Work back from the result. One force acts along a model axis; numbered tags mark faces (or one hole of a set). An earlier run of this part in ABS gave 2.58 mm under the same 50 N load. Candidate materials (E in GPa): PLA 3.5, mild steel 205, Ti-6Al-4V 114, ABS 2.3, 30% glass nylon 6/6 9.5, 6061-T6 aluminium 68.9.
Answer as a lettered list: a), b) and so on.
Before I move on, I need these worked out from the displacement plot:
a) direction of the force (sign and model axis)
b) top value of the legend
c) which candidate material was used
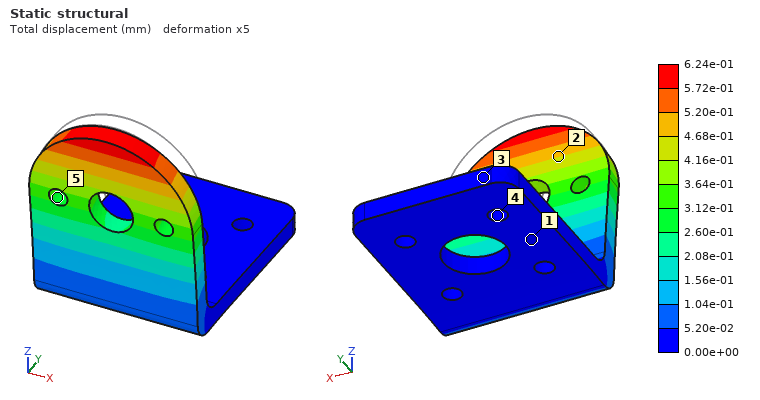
a) -Y
b) 6.24e-01 mm
c) 30% glass nylon 6/6
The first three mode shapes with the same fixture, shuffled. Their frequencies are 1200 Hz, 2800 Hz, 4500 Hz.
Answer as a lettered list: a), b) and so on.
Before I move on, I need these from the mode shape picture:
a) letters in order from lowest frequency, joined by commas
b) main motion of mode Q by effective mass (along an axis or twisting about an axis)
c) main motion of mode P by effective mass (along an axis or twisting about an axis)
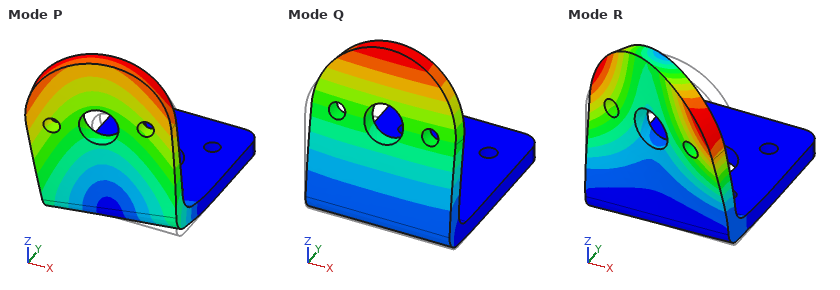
a) Q, P, R
b) along Y
c) along X
